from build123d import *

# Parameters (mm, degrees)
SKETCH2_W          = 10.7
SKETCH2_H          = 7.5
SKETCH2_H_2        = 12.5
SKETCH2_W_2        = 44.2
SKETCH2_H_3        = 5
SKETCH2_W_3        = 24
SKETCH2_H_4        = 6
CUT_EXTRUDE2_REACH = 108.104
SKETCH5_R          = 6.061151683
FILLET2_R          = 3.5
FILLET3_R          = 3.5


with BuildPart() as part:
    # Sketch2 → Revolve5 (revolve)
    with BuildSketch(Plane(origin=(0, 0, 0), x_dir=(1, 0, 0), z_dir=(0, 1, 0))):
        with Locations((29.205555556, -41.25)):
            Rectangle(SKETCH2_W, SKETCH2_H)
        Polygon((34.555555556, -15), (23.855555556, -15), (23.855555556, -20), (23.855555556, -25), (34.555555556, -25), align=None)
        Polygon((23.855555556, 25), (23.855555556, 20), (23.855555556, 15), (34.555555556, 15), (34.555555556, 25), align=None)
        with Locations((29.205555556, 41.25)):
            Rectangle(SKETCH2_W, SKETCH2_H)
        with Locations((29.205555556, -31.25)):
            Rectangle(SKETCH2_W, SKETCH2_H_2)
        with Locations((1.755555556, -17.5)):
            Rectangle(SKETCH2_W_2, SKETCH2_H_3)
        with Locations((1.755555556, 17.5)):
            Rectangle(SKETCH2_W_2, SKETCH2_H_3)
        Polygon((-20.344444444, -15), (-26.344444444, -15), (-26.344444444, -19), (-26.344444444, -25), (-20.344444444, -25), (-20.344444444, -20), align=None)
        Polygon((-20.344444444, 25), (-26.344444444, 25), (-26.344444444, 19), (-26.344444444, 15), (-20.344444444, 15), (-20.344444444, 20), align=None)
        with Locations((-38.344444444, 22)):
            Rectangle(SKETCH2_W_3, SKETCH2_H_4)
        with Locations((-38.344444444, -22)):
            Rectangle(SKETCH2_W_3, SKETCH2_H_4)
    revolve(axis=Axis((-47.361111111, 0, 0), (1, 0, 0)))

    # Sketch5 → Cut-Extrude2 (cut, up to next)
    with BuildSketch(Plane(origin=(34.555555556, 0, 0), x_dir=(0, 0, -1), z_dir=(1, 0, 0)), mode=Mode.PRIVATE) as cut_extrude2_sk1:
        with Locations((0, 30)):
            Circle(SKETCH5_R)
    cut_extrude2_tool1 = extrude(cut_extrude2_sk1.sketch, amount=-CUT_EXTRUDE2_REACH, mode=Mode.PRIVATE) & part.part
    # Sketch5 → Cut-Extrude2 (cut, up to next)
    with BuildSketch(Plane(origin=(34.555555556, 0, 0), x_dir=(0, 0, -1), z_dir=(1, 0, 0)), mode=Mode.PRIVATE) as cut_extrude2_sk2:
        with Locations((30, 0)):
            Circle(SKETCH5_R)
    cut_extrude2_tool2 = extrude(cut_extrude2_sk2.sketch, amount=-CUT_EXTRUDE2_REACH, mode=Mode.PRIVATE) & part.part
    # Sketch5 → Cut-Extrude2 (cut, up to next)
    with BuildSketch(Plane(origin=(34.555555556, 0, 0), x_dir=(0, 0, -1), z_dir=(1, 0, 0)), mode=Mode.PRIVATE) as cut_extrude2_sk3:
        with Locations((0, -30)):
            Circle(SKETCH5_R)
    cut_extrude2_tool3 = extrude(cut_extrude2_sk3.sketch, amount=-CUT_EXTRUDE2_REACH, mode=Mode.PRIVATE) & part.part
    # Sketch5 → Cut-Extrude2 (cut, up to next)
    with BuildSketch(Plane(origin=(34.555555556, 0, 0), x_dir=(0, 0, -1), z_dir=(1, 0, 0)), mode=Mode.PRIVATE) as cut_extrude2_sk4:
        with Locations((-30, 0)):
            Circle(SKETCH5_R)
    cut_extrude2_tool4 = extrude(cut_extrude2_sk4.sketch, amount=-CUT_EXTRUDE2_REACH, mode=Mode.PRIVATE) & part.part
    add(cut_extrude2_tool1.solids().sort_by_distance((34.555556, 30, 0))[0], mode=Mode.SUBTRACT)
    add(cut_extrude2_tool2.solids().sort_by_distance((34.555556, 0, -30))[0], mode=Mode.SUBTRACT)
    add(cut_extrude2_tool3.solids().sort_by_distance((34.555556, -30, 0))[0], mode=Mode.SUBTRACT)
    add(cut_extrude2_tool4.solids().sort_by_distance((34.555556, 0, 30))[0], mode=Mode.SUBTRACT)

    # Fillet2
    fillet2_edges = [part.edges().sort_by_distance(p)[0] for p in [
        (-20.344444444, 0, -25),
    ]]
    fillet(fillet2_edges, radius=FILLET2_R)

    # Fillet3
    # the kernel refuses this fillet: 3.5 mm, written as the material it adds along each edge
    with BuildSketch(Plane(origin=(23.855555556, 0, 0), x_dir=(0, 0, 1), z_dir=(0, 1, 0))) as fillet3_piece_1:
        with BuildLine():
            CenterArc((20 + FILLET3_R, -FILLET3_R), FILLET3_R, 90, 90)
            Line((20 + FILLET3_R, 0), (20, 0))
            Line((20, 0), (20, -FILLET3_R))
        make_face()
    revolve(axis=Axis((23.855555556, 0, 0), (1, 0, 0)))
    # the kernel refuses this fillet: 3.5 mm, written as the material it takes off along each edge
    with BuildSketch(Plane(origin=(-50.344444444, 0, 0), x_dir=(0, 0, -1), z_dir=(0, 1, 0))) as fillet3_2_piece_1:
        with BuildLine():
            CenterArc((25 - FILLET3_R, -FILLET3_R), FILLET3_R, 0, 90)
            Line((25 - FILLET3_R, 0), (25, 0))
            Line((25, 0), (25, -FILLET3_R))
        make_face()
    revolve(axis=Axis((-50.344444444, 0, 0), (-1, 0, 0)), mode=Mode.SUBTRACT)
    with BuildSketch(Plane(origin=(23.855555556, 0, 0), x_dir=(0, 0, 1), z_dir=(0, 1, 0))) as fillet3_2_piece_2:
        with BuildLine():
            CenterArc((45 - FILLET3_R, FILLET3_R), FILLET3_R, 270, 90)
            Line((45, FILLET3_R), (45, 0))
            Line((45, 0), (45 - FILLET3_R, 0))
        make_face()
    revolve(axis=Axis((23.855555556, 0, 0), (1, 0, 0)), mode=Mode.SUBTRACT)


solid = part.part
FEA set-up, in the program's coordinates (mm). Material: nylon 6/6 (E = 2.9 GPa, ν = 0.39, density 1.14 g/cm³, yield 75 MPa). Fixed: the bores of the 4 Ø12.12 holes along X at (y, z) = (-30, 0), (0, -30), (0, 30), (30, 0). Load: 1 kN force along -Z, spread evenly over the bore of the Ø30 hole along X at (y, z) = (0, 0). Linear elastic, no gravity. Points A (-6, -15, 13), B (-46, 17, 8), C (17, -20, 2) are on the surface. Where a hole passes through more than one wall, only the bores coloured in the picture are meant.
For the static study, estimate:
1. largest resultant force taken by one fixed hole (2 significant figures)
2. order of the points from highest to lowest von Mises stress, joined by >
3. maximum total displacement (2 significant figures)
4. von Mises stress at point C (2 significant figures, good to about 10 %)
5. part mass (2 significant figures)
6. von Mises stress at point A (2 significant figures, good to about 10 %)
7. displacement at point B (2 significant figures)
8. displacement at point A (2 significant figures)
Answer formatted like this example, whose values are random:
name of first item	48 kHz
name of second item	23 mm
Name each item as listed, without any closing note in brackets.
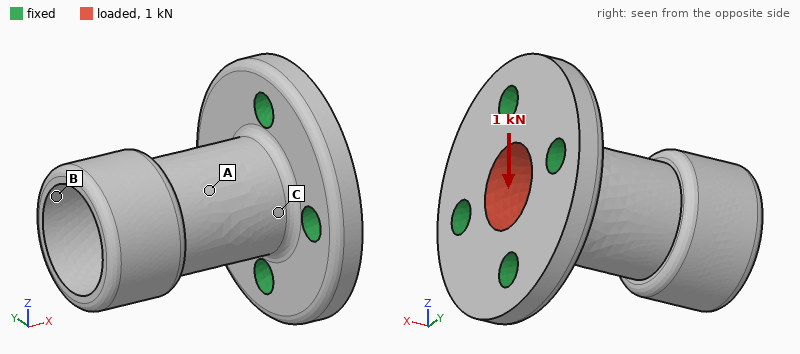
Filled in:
largest resultant force taken by one fixed hole	570 N
order of the points from highest to lowest von Mises stress, joined by >	C > A > B
maximum total displacement	0.22 mm
von Mises stress at point C	2.5 MPa
part mass	120 g
von Mises stress at point A	1.5 MPa
displacement at point B	0.20 mm
displacement at point A	0.11 mm
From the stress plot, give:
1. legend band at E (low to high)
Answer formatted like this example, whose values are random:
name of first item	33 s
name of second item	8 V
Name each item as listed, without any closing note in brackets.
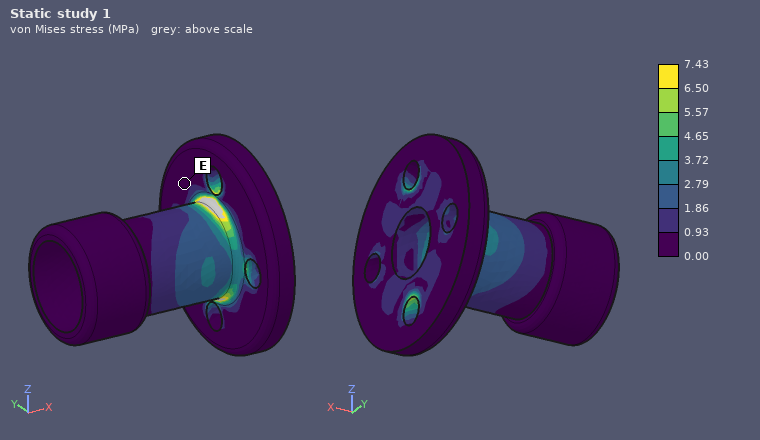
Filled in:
legend band at E	0.00 to 0.93 MPa
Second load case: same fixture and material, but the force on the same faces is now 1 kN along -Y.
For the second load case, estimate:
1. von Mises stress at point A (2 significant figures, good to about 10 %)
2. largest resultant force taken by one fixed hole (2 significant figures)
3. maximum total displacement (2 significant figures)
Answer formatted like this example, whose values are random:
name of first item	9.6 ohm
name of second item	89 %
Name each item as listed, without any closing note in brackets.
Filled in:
von Mises stress at point A	1.4 MPa
largest resultant force taken by one fixed hole	570 N
maximum total displacement	0.22 mm
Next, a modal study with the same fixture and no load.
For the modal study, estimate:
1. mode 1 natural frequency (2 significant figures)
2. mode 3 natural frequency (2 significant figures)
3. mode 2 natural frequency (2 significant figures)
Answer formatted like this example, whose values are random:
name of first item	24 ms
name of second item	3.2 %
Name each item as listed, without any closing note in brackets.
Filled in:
mode 1 natural frequency	1100 Hz
mode 3 natural frequency	2300 Hz
mode 2 natural frequency	1100 Hz
